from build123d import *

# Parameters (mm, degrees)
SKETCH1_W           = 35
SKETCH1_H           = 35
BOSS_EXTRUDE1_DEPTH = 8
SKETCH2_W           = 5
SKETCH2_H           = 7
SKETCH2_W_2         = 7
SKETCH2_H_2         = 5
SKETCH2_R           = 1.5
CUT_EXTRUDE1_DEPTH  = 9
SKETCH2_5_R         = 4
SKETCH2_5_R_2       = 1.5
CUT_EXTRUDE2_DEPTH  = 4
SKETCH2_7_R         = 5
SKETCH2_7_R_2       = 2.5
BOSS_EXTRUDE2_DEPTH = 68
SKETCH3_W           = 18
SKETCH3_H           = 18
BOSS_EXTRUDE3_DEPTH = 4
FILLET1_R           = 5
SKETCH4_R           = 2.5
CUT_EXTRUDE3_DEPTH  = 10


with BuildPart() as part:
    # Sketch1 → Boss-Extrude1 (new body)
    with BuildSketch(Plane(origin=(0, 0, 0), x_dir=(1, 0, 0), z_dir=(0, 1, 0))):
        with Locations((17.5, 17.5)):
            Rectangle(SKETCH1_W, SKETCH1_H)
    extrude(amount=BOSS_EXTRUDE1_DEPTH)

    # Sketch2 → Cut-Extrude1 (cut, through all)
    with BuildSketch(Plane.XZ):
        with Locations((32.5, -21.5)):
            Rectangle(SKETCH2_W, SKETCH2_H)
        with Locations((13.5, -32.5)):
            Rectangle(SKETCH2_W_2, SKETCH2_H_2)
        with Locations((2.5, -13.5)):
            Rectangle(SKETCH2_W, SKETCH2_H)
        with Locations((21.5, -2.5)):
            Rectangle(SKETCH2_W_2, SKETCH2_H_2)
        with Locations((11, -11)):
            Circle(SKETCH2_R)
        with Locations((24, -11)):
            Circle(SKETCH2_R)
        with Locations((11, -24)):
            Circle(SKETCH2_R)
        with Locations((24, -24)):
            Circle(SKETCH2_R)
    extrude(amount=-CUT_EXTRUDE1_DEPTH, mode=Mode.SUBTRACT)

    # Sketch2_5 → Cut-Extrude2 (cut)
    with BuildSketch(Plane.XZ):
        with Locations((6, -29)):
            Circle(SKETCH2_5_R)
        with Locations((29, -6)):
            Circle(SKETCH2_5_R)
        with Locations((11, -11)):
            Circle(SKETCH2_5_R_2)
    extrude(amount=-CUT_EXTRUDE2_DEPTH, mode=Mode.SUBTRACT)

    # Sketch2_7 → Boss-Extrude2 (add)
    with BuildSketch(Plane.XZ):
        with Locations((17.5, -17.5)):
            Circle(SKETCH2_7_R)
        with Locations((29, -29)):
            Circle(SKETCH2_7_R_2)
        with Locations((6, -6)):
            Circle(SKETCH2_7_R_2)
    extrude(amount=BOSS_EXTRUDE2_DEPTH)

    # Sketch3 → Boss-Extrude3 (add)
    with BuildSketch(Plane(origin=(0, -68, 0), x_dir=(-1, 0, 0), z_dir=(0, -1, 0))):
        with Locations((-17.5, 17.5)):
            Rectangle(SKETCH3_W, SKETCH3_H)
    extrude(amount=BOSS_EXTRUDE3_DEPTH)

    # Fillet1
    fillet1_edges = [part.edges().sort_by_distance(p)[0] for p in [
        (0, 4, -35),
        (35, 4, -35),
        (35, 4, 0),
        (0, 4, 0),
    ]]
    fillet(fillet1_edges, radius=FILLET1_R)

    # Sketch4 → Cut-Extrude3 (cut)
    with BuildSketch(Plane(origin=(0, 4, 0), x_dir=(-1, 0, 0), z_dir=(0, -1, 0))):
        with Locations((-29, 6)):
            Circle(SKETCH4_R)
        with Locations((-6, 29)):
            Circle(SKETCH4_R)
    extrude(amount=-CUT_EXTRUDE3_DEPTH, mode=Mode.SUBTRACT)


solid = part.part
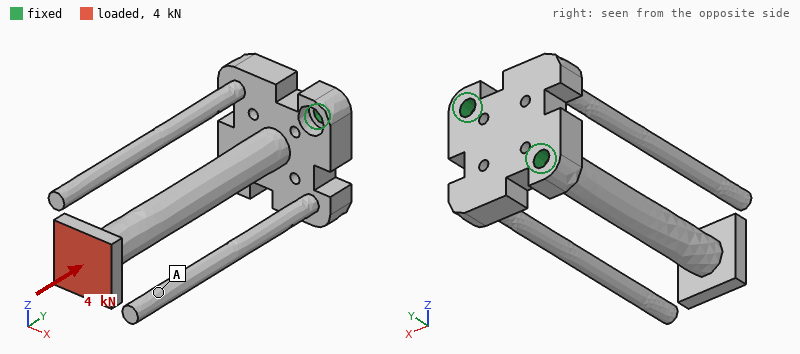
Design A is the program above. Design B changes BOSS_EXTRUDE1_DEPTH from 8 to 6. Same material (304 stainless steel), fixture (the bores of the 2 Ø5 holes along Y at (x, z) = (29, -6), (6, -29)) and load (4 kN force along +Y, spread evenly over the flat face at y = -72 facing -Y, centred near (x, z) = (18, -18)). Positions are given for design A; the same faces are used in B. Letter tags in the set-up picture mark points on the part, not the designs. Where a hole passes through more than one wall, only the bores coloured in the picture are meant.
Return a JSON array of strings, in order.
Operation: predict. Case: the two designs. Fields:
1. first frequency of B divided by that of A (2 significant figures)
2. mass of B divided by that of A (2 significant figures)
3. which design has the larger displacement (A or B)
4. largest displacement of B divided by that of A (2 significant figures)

["0.85", "0.88", "B", "1.3"]
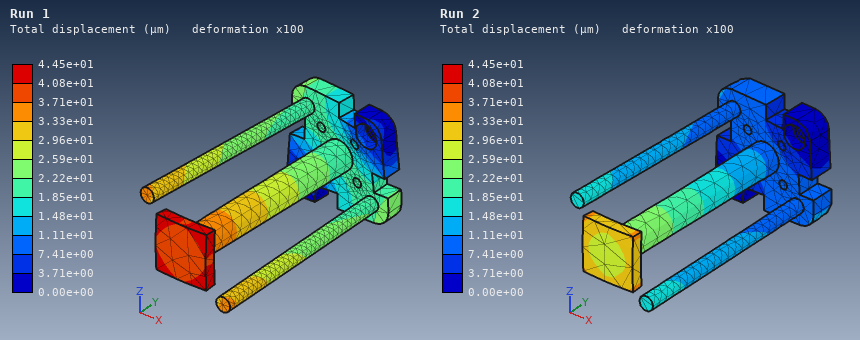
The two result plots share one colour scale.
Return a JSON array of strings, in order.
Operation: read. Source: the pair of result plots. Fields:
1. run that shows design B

["Run 1"]
